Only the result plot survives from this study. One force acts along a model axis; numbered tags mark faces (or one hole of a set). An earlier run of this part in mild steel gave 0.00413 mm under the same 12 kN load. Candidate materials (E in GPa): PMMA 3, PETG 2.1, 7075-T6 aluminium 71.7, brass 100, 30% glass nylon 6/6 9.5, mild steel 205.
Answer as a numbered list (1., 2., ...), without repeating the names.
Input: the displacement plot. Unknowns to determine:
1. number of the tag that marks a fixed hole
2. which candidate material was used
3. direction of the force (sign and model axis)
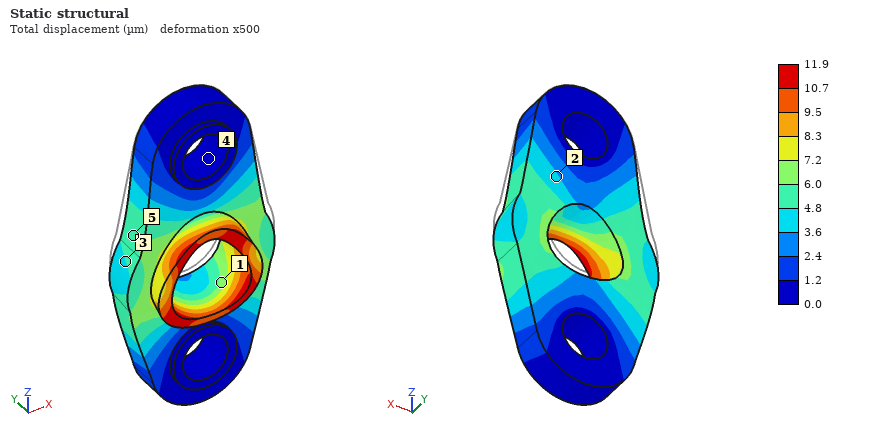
1. 4
2. 7075-T6 aluminium
3. -Z
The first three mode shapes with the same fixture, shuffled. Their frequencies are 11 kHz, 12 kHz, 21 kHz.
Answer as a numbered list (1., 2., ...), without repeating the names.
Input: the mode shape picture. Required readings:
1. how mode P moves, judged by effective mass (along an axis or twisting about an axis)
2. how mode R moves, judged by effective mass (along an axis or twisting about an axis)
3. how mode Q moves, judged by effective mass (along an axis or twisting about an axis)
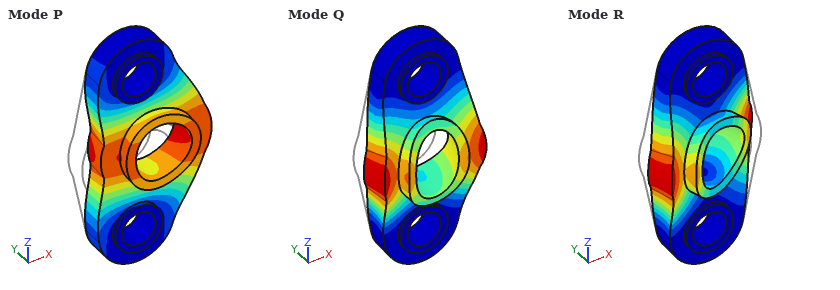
1. along X
2. twisting about Z
3. along Y
